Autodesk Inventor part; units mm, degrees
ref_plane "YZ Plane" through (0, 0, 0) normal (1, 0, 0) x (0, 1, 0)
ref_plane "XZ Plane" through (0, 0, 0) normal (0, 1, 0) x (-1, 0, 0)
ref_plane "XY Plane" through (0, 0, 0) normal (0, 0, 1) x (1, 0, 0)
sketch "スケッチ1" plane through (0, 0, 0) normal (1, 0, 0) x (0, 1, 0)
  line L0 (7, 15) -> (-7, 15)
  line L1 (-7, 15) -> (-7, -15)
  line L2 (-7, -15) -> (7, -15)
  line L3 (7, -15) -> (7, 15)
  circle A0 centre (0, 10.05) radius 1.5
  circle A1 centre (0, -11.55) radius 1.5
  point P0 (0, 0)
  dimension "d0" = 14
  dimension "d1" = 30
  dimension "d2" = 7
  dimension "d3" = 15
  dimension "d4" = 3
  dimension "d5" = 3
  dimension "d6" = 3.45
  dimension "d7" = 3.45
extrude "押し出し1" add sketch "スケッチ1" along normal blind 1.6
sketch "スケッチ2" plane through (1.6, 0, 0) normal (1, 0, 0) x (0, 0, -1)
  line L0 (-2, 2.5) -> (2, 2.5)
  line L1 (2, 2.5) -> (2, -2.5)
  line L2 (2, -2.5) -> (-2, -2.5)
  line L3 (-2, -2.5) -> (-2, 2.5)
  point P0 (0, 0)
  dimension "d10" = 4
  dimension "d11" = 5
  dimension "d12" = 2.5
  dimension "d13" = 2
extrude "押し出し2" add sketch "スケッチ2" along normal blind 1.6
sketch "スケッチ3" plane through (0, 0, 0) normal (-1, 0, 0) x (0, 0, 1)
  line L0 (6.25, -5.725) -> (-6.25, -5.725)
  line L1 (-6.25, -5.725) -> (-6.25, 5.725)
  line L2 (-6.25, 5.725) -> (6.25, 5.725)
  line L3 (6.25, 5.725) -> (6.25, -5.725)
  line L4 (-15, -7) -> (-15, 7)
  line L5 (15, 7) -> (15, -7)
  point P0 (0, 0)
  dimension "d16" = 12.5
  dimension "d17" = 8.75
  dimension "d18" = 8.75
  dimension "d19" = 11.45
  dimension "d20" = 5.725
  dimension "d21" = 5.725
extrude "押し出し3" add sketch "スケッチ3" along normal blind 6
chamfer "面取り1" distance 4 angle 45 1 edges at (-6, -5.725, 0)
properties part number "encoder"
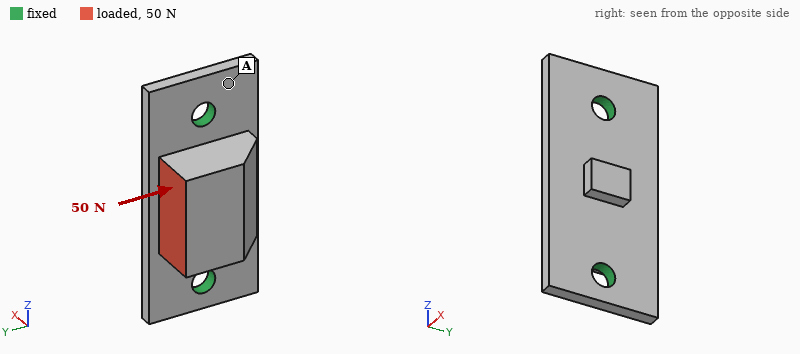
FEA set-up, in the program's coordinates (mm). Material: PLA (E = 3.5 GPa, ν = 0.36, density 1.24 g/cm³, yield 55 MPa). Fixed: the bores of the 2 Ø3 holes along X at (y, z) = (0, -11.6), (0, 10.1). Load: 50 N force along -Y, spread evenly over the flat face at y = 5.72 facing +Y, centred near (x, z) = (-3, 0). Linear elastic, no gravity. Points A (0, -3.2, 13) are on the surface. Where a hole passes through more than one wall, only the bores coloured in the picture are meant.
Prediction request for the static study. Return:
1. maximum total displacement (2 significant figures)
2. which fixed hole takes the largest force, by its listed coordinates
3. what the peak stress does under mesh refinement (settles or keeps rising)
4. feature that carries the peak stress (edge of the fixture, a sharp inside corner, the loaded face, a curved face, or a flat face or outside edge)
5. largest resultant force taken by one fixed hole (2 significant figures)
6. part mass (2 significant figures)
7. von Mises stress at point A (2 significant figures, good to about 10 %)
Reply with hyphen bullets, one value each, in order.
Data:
- 0.11 mm
- (0, 10.1)
- keeps rising
- edge of the fixture
- 27 N
- 1.8 g
- 4.5 MPa
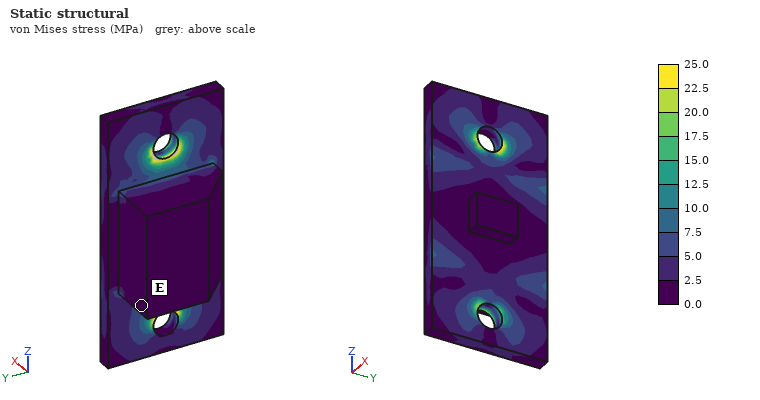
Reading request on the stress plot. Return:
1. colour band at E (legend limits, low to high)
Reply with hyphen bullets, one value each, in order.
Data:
- 0.0 to 2.5 MPa
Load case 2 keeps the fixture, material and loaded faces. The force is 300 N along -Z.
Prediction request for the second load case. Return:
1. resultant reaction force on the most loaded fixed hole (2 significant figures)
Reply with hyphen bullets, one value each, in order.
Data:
- 190 N
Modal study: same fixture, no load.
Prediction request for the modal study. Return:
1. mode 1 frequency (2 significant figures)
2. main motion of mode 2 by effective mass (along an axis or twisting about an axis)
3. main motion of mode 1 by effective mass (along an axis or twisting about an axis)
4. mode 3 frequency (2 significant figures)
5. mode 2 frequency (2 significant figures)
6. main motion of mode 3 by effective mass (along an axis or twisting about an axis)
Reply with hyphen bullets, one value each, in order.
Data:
- 3600 Hz
- along X
- along Y
- 10 kHz
- 5800 Hz
- along Z
